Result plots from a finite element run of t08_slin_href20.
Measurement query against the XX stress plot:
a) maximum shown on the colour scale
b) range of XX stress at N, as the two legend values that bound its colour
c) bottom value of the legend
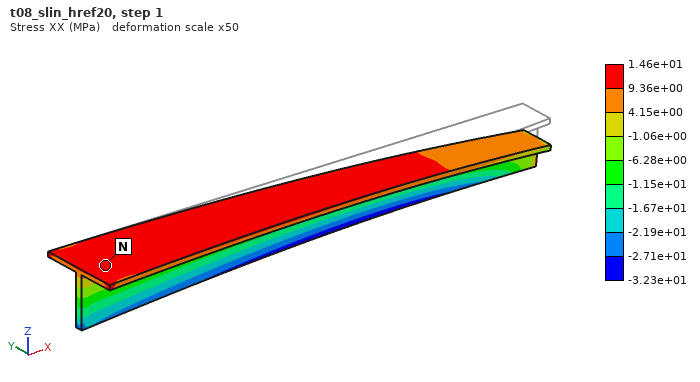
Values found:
1.46e+01 MPa
9.36e+00 to 1.46e+01 MPa
-3.23e+01 MPa
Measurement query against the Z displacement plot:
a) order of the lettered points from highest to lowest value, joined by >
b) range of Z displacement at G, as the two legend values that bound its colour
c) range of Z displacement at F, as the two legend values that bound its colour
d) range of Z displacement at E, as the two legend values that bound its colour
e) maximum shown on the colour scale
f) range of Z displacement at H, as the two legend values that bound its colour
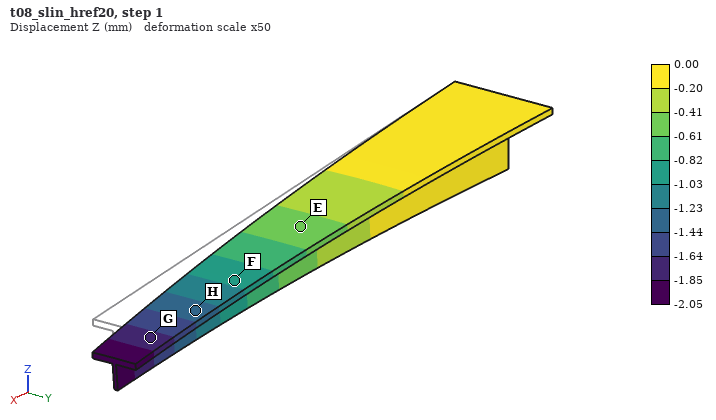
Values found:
E > F > H > G
-1.85 to -1.64 mm
-1.03 to -0.82 mm
-0.61 to -0.41 mm
0.00 mm
-1.44 to -1.23 mm
